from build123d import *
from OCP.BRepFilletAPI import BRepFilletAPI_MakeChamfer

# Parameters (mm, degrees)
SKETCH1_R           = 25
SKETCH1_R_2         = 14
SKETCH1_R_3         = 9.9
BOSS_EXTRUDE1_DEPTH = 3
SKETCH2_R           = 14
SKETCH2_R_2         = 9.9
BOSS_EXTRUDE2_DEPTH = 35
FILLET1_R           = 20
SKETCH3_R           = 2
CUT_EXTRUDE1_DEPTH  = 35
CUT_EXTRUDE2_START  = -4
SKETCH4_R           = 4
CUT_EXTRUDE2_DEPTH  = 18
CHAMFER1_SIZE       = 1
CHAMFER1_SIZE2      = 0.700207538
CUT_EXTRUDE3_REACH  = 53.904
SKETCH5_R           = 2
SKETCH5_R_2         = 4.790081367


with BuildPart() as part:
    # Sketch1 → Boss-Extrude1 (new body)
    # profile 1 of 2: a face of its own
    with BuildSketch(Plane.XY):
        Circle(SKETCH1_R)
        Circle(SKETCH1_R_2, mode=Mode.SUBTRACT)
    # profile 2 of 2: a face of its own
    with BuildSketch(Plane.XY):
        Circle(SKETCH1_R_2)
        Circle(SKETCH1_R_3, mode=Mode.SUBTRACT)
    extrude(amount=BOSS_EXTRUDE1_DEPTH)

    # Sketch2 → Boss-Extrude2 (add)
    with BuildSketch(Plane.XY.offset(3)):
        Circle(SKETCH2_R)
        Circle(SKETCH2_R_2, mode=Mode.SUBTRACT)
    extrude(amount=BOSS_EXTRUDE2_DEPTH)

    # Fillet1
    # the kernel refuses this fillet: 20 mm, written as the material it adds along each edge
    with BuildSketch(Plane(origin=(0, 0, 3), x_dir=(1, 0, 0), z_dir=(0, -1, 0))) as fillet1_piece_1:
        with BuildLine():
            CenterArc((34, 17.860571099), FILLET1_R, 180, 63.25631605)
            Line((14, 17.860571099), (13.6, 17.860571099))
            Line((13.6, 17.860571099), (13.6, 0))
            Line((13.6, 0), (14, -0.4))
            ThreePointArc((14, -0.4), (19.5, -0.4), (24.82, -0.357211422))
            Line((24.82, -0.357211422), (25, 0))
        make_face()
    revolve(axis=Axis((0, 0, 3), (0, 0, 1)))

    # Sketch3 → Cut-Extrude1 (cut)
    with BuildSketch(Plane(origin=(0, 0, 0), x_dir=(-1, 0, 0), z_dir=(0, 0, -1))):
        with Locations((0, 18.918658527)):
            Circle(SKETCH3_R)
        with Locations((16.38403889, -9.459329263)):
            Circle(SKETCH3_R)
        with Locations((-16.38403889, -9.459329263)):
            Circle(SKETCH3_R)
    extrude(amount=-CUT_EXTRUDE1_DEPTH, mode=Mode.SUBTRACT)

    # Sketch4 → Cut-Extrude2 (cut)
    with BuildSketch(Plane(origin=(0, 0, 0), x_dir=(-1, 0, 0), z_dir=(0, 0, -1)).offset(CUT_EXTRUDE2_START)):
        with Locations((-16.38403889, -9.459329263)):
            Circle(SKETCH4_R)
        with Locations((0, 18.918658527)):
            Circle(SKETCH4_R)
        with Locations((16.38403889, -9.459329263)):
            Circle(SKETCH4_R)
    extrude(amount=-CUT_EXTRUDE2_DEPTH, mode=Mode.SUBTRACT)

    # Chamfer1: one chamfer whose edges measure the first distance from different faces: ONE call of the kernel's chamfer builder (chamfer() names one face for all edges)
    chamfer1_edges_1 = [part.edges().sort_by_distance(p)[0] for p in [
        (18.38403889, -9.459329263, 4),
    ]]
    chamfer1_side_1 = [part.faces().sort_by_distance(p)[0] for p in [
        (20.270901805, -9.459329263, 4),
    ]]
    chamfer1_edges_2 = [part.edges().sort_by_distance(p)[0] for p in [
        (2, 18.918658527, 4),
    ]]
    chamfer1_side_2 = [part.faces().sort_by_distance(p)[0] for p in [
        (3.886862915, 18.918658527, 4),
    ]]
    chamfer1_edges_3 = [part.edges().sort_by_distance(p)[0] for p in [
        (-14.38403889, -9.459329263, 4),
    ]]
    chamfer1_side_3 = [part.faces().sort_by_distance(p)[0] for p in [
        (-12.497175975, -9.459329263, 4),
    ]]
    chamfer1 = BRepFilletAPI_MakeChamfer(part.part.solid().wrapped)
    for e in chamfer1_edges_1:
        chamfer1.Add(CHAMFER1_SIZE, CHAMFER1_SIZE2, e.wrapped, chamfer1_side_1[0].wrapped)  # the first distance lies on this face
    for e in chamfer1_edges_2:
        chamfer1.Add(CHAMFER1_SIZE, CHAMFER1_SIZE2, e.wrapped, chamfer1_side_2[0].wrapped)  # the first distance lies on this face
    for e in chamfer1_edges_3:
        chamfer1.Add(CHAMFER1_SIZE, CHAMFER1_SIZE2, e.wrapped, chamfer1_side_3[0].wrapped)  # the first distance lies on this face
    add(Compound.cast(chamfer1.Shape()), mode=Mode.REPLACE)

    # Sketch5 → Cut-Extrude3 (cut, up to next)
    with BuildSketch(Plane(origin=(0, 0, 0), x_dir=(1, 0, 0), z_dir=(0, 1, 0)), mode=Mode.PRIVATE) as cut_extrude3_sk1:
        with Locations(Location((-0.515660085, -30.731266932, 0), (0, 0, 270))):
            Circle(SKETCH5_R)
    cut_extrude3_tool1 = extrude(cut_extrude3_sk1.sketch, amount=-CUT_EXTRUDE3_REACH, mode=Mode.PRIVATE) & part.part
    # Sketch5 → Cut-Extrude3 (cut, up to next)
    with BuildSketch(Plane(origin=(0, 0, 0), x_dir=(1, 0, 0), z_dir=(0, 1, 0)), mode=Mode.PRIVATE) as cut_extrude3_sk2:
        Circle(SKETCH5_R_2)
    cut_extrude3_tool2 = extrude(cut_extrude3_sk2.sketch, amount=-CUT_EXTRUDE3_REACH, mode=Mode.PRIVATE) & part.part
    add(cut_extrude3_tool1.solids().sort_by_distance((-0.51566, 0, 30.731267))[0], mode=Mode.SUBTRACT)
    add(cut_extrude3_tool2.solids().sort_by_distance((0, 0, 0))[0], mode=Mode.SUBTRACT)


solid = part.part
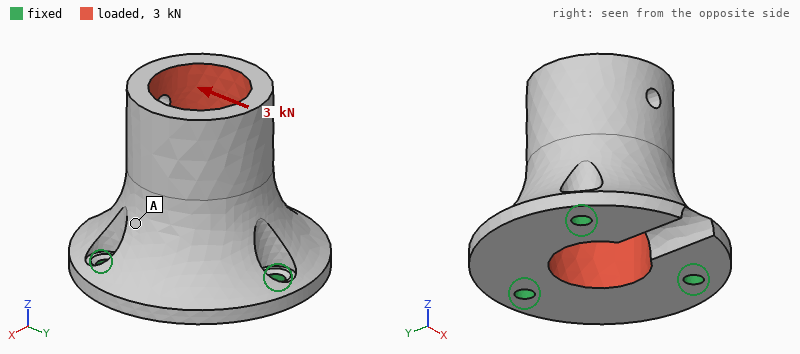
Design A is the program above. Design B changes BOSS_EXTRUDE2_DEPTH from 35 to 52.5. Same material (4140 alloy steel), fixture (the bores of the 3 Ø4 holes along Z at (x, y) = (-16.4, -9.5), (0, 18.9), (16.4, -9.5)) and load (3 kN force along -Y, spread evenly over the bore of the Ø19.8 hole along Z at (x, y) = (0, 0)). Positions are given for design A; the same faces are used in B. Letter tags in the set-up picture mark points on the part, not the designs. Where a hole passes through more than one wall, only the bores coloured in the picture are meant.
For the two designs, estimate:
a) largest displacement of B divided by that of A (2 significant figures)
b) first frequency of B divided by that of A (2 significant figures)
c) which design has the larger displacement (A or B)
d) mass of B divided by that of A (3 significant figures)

2.2
0.58
B
1.26
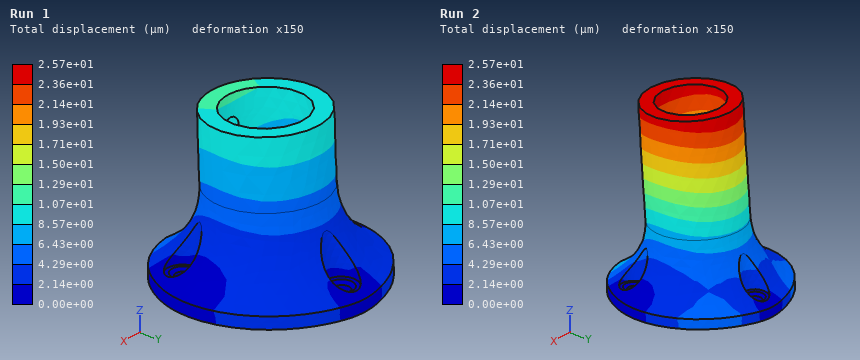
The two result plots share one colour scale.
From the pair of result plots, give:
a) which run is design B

Run 2
